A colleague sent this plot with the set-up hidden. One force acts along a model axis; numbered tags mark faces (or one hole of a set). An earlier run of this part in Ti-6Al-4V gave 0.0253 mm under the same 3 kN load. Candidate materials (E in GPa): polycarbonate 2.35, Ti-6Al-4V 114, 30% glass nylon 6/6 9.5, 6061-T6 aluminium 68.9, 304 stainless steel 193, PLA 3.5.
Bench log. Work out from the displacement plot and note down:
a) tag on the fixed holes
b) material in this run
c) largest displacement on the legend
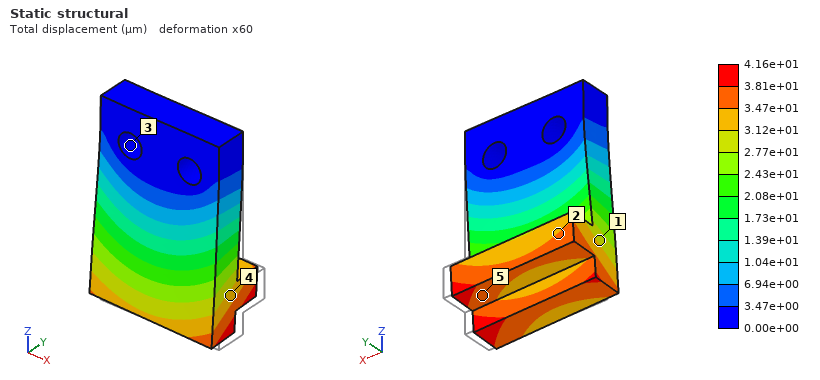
3
6061-T6 aluminium
4.16e+01 µm
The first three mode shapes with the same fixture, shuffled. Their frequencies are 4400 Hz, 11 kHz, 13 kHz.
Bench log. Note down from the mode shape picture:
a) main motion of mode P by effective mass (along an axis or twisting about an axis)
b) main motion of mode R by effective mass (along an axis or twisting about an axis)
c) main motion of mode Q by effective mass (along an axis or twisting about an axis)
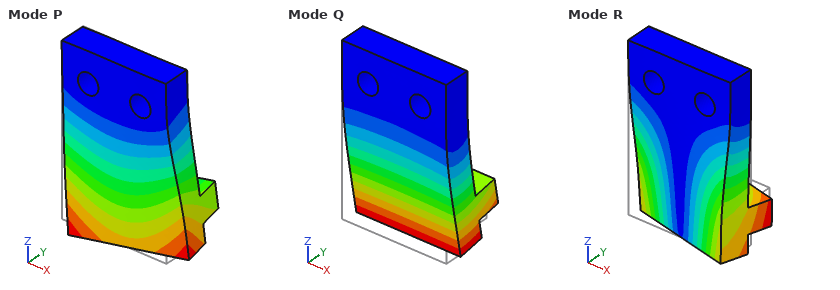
along X
along X
along Y
